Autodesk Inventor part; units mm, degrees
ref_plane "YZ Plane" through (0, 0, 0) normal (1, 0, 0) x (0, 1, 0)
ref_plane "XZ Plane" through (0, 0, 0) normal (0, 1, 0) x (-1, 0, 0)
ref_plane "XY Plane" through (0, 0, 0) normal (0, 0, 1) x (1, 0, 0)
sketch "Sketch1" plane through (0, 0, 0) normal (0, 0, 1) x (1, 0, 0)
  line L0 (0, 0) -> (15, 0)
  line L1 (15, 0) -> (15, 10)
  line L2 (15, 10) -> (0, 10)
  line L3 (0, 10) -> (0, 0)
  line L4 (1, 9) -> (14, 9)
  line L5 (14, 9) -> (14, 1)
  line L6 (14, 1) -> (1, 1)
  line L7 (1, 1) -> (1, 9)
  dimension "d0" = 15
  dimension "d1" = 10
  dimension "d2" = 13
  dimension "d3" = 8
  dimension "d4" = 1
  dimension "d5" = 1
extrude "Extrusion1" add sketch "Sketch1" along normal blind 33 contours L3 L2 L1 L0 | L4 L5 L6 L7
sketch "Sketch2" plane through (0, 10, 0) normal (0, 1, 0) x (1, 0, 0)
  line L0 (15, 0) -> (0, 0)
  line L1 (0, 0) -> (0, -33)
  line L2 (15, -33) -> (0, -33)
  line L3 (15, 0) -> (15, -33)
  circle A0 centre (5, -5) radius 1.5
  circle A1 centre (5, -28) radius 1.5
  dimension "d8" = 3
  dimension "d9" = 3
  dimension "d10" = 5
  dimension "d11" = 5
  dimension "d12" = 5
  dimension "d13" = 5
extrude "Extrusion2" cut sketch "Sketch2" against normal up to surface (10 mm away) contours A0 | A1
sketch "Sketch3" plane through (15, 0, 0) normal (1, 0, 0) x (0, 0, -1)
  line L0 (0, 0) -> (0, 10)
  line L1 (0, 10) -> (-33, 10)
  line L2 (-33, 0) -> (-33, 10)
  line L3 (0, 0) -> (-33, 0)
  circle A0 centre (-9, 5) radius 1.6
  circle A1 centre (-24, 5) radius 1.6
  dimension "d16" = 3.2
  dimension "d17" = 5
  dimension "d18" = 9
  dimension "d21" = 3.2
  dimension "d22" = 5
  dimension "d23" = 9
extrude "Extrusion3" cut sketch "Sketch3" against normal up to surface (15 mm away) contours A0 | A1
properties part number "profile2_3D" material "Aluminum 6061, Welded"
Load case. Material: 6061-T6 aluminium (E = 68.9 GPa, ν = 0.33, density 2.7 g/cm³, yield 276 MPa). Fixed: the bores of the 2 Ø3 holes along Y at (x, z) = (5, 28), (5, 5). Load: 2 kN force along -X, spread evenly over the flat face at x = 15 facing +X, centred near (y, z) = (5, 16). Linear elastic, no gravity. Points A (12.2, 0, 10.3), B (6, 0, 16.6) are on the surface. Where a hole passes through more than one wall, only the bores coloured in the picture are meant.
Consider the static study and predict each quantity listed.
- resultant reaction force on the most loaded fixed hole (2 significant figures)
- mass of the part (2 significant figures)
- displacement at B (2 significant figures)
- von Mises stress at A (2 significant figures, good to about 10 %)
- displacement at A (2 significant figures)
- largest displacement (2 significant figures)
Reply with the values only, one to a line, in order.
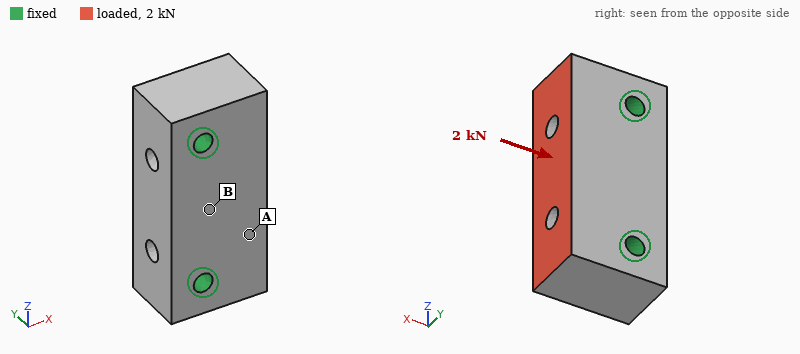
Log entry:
1.0 kN
12 g
2.0 µm
7.4 MPa
1.7 µm
2.4 µm
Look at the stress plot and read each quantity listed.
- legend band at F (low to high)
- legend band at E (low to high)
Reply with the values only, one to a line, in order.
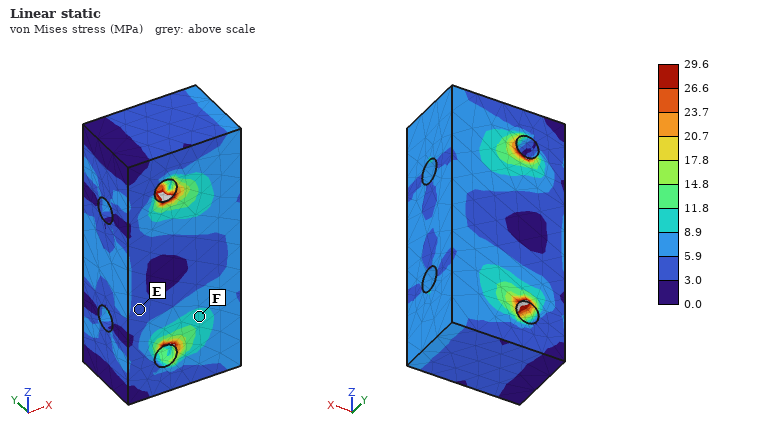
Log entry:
8.9 to 11.8 MPa
3.0 to 5.9 MPa
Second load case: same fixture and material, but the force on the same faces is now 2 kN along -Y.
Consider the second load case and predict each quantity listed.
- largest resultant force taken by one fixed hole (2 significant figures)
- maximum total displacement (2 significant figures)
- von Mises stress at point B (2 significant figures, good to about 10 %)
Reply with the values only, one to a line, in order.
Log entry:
1.0 kN
15 µm
10 MPa
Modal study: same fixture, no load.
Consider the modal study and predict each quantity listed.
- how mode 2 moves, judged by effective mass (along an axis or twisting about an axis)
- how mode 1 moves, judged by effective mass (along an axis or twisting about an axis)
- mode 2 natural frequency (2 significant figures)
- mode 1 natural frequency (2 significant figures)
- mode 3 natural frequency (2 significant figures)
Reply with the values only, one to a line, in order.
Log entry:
along X
along Y
46 kHz
35 kHz
49 kHz
